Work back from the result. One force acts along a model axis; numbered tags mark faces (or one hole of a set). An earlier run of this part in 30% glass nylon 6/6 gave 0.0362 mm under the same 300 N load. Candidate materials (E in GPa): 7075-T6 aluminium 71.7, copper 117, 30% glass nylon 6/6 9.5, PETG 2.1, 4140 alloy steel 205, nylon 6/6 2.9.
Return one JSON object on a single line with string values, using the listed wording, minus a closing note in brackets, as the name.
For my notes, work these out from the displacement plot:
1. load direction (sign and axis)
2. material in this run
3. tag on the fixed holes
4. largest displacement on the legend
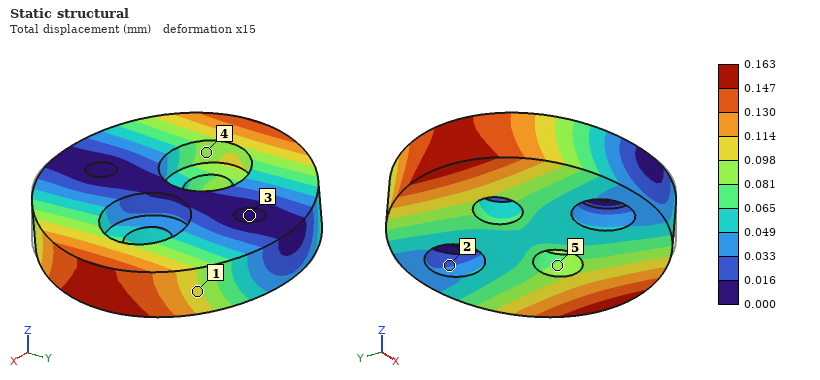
{"load direction": "-X", "material in this run": "PETG", "tag on the fixed holes": "3", "largest displacement on the legend": "0.163 mm"}
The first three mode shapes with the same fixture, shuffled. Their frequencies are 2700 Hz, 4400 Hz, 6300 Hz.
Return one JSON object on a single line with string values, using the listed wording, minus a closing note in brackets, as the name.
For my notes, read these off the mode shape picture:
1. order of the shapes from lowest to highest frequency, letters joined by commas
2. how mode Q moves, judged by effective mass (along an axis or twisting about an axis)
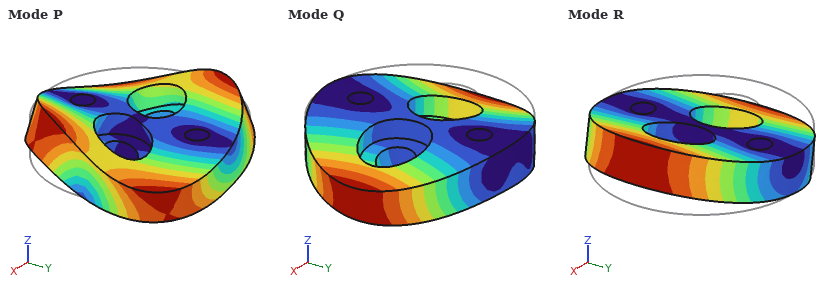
{"order of the shapes from lowest to highest frequency, letters joined by commas": "R, Q, P", "how mode Q moves, judged by effective mass": "along Z"}
